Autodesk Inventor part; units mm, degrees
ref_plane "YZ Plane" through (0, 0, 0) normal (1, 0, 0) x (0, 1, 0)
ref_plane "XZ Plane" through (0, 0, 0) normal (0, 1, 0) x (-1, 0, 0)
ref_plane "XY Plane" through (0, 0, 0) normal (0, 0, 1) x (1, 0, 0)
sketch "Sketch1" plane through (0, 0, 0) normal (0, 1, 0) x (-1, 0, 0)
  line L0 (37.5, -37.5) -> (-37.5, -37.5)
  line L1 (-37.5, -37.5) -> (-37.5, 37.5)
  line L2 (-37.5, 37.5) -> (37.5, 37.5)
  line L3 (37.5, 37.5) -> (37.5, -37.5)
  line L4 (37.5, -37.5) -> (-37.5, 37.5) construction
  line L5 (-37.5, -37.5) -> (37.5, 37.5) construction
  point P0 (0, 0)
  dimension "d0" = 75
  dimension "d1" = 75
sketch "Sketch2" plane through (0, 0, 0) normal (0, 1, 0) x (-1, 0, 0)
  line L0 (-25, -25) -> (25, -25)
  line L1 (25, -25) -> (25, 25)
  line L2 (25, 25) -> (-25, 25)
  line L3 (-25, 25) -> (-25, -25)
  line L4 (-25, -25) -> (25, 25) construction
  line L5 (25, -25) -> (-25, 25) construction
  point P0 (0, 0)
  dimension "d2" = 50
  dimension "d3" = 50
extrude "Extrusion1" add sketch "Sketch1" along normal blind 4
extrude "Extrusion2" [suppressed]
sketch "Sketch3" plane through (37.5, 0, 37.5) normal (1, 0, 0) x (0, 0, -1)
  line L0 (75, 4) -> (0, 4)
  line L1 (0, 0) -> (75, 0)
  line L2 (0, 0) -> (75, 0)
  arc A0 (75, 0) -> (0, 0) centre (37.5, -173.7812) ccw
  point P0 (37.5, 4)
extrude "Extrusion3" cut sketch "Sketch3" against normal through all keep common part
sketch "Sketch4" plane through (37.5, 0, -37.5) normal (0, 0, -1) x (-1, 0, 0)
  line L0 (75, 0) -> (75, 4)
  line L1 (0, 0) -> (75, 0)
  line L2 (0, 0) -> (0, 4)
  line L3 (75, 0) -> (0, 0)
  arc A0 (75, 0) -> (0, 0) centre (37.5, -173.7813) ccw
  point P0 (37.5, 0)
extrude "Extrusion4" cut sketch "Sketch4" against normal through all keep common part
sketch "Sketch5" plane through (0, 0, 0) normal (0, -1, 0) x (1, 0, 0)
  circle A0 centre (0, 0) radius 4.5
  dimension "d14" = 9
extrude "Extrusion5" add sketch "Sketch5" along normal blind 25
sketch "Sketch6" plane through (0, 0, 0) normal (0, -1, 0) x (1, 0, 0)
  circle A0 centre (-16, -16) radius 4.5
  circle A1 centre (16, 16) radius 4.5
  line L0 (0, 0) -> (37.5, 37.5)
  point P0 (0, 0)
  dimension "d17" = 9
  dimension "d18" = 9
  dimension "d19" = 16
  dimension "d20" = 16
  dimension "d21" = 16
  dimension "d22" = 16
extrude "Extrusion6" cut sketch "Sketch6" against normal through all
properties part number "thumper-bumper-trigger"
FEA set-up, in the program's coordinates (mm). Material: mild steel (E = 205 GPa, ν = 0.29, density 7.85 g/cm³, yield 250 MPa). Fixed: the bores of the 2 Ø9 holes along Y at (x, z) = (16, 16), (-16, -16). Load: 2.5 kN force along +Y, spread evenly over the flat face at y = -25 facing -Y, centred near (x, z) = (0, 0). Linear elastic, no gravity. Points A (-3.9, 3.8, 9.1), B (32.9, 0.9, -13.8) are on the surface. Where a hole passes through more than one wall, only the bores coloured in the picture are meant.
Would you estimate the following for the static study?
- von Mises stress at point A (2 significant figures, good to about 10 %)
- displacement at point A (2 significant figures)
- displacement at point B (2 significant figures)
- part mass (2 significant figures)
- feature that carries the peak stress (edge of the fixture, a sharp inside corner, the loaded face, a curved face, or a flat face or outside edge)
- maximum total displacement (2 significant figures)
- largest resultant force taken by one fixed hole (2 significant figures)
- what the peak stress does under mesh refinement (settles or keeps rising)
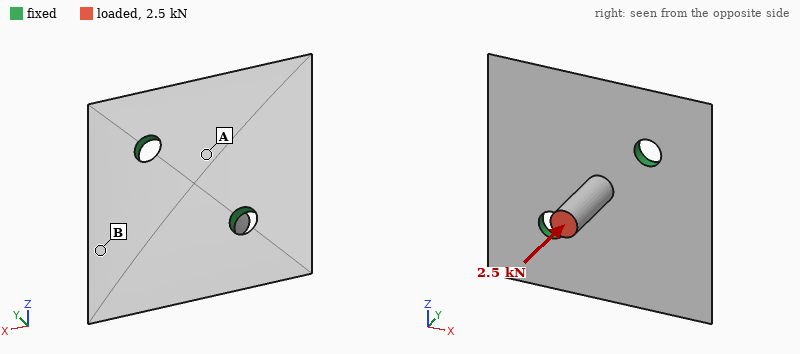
86 MPa
29 µm
26 µm
98 g
edge of the fixture
41 µm
1.3 kN
keeps rising
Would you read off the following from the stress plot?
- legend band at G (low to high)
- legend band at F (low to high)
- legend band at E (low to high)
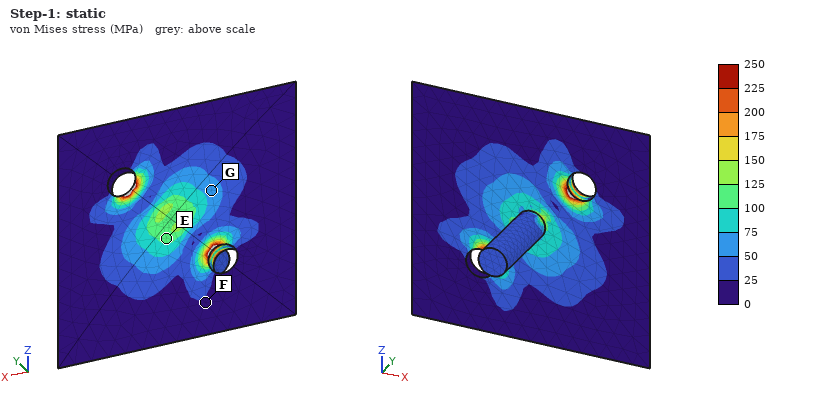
50 to 75 MPa
0 to 25 MPa
100 to 125 MPa
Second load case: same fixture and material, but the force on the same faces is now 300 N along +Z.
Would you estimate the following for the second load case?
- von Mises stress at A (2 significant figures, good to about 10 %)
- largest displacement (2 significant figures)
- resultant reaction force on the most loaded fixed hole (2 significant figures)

31 MPa
64 µm
250 N
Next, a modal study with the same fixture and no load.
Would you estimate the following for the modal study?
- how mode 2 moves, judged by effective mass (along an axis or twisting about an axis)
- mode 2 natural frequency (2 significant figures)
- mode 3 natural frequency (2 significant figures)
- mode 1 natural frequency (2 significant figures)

along Y
2700 Hz
5400 Hz
2100 Hz
